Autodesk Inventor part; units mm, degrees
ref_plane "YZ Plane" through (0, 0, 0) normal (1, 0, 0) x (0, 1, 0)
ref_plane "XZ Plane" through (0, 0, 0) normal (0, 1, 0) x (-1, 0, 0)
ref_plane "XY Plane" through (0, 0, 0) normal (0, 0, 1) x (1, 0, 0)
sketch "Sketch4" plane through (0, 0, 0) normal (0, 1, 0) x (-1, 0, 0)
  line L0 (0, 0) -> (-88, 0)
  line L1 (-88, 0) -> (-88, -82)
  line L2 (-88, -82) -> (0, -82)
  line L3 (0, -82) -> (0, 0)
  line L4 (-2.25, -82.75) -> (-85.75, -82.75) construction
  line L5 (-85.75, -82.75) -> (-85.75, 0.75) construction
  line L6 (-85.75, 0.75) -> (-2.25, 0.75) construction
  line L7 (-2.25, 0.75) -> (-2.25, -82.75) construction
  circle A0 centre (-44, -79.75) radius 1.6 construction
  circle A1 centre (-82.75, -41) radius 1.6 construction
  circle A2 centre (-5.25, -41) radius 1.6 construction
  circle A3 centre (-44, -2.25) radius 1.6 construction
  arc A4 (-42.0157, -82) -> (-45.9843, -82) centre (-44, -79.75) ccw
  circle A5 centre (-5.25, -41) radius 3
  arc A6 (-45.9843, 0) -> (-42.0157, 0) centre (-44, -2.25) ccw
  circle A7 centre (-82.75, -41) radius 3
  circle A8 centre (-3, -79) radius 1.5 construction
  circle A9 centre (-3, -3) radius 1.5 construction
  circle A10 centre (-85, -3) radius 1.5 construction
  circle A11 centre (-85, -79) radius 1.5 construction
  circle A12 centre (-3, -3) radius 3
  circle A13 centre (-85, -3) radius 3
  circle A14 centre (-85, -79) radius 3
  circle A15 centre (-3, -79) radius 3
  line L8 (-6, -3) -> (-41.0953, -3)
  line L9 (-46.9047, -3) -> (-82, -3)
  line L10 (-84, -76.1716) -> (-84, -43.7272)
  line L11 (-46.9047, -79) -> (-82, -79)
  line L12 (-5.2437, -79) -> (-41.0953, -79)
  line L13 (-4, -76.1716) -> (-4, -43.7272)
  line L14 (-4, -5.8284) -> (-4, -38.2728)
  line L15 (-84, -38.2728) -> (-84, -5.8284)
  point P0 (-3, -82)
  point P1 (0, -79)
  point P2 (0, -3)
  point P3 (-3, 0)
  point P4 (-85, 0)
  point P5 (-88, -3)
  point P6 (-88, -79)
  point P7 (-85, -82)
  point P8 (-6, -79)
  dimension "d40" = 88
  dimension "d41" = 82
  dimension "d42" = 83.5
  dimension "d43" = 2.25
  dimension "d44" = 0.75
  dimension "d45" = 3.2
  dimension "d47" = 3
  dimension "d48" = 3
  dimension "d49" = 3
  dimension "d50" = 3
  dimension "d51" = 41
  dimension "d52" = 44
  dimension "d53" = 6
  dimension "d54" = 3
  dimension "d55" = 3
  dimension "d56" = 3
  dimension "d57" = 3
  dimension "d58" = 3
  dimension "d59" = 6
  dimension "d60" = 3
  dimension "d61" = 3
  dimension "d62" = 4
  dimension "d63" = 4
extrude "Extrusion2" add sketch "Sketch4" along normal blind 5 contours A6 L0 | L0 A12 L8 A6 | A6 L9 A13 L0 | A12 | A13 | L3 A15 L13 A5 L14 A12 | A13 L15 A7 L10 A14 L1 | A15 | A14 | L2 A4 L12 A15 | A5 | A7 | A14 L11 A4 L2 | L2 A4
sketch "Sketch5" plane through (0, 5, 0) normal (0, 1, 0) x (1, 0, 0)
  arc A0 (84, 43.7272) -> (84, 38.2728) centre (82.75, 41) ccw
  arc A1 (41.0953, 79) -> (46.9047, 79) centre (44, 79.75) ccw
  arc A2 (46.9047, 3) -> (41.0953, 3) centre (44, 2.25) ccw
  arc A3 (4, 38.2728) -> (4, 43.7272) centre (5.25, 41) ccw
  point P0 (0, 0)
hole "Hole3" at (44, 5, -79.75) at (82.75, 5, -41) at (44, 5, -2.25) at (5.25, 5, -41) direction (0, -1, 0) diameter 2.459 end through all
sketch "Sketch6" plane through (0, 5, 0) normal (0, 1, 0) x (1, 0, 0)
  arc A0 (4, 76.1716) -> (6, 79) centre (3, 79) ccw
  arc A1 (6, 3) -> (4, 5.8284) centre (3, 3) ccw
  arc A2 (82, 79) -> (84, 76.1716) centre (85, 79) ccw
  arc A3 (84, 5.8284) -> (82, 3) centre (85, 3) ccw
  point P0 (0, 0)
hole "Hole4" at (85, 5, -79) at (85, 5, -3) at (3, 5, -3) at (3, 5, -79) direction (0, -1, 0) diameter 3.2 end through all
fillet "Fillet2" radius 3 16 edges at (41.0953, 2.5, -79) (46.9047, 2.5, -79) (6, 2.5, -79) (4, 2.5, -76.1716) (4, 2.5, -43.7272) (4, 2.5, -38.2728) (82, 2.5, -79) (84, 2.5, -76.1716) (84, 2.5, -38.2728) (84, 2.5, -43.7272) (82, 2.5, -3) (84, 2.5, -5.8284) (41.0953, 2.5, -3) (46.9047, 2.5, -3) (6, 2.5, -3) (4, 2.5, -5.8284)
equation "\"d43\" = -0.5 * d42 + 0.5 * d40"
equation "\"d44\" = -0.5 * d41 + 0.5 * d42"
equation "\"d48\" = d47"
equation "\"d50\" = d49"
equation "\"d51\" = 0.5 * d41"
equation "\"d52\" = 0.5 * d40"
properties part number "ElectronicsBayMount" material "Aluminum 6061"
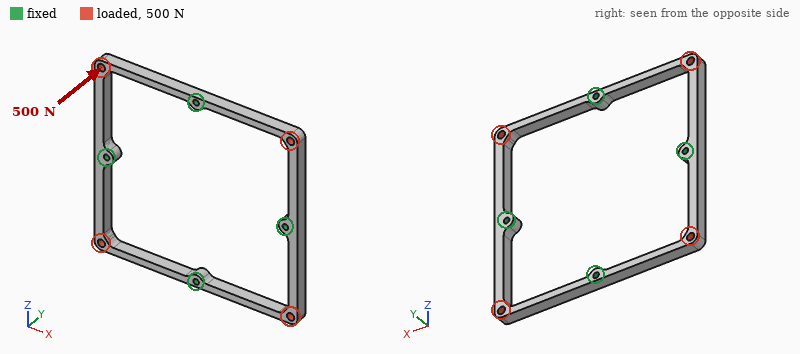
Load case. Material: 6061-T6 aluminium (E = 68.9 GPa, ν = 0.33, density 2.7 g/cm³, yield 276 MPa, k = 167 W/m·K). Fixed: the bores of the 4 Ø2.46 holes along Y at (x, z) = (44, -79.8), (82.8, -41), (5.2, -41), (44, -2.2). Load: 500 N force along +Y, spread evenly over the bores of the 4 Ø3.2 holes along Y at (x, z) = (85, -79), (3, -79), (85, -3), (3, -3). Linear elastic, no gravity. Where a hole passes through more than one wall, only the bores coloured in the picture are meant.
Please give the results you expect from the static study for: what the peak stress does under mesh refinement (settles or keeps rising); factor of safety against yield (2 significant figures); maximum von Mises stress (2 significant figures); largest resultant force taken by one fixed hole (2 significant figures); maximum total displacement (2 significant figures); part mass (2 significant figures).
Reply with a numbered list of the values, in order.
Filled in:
1. settles
2. 1.7
3. 170 MPa
4. 140 N
5. 0.37 mm
6. 16 g
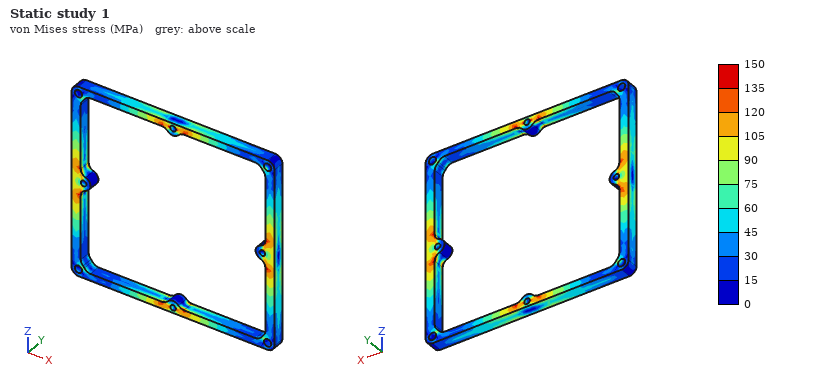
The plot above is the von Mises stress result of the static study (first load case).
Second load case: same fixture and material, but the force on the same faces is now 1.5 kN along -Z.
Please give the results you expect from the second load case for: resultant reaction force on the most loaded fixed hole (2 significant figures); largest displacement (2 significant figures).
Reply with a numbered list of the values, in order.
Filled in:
1. 740 N
2. 22 µm
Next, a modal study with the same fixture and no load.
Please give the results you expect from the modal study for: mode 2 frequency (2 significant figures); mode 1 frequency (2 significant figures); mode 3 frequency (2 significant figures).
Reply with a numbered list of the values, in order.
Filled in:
1. 2900 Hz
2. 2900 Hz
3. 3000 Hz
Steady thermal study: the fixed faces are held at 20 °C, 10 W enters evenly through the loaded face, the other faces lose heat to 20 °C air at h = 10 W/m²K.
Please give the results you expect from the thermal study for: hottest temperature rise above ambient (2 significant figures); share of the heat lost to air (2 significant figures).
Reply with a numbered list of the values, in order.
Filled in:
1. 16 K
2. 4.3 %
